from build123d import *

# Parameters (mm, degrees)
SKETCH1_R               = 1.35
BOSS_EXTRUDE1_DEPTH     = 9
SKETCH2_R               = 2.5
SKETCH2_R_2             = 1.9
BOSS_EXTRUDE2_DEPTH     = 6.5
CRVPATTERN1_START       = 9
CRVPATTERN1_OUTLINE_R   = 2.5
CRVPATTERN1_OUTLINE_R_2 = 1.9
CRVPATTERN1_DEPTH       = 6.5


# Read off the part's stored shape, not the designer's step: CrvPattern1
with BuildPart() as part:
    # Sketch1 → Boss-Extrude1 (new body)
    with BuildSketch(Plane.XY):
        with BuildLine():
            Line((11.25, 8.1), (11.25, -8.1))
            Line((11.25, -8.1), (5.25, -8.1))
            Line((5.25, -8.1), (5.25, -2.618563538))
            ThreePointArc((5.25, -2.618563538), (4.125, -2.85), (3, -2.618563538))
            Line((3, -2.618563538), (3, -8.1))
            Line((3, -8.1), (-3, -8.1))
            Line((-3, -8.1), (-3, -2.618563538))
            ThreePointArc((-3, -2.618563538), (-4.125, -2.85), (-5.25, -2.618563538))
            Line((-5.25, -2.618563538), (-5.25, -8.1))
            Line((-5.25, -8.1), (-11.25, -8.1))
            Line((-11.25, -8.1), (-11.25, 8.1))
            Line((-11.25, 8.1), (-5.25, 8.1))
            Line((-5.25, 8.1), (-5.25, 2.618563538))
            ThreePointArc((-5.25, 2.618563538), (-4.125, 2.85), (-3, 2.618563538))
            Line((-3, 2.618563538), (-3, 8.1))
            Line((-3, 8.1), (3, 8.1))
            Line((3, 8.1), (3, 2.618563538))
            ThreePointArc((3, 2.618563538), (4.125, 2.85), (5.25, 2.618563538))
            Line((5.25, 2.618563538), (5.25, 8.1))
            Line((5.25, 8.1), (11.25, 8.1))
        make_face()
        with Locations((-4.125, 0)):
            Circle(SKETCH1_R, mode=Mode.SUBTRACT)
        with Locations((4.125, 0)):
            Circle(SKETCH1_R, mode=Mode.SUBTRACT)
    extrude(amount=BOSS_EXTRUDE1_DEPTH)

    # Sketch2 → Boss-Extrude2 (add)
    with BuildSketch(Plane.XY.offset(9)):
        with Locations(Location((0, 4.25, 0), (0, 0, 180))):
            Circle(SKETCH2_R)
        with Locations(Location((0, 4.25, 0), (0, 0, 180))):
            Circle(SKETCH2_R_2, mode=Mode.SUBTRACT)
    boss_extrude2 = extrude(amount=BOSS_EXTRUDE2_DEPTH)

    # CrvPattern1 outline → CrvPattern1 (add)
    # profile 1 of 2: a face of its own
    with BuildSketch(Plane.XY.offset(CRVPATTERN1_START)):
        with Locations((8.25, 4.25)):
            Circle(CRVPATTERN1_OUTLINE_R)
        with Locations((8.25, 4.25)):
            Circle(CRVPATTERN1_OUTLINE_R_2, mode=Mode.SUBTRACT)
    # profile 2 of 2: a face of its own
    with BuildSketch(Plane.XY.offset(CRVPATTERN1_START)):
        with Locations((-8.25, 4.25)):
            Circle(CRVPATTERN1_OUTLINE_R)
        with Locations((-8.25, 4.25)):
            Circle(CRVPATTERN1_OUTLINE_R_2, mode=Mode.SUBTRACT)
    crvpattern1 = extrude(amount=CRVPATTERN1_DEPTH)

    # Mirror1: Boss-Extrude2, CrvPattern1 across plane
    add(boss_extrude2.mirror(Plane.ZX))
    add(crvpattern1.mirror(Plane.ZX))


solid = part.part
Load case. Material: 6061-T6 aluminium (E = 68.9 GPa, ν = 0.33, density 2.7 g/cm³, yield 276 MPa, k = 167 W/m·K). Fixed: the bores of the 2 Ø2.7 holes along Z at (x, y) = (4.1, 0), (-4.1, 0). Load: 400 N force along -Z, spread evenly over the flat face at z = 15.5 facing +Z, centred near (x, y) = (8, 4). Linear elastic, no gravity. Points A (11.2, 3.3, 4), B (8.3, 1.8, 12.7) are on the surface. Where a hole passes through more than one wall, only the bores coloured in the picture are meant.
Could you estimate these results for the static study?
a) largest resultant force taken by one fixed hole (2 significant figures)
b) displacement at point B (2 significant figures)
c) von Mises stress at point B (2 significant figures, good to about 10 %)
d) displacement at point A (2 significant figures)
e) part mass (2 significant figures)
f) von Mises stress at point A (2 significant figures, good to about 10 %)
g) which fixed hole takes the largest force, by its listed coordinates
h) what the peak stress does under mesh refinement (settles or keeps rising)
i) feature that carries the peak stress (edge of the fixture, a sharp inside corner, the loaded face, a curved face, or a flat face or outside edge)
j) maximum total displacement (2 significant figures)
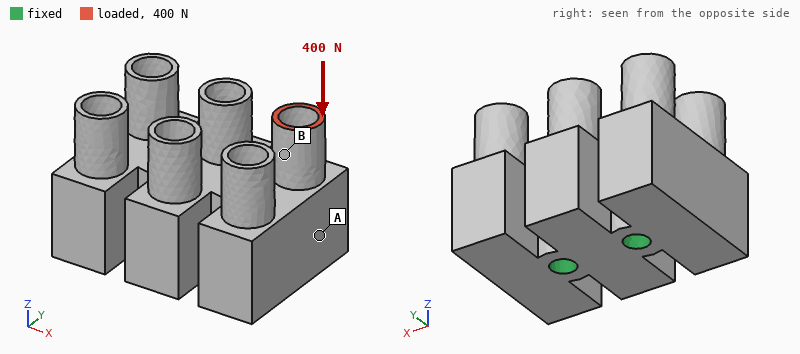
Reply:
400 N
5.6 µm
49 MPa
2.6 µm
8.3 g
7.7 MPa
(4.1, 0)
keeps rising
edge of the fixture
10 µm
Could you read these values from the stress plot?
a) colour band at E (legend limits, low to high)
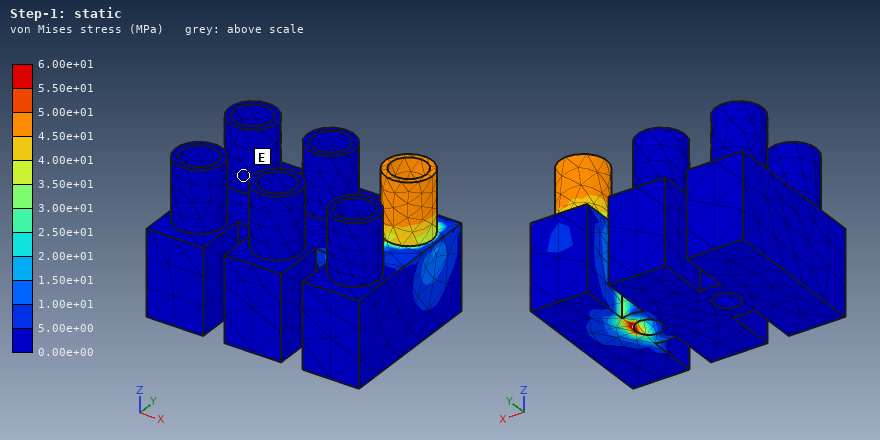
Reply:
0.00e+00 to 5.00e+00 MPa
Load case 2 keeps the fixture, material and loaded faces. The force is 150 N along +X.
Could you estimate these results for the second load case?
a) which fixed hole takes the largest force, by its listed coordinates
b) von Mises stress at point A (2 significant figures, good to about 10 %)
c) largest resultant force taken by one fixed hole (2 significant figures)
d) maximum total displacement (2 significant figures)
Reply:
(4.1, 0)
17 MPa
140 N
34 µm
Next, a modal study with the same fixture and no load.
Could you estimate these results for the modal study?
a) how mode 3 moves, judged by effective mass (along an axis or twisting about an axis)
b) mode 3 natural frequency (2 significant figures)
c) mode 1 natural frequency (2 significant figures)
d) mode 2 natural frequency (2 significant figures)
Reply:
twisting about X
38 kHz
25 kHz
26 kHz
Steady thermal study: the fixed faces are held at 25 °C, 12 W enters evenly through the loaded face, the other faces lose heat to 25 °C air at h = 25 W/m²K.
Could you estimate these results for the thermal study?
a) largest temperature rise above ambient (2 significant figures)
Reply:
68 K
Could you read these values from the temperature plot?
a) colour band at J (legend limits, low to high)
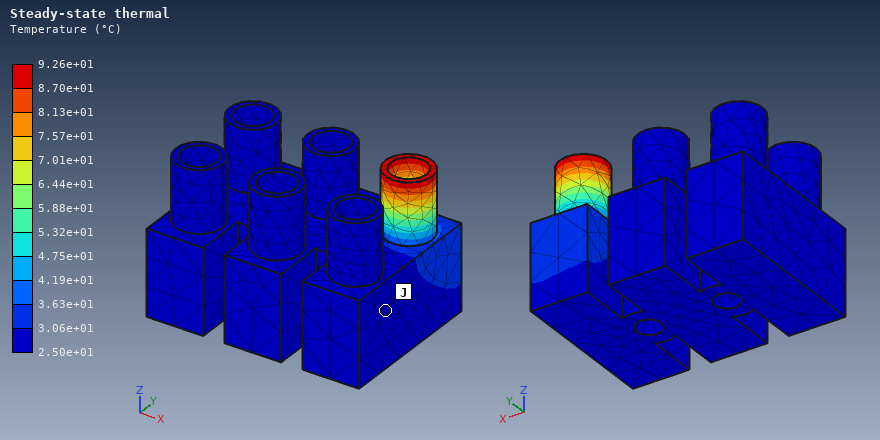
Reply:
2.50e+01 to 3.06e+01 °C
